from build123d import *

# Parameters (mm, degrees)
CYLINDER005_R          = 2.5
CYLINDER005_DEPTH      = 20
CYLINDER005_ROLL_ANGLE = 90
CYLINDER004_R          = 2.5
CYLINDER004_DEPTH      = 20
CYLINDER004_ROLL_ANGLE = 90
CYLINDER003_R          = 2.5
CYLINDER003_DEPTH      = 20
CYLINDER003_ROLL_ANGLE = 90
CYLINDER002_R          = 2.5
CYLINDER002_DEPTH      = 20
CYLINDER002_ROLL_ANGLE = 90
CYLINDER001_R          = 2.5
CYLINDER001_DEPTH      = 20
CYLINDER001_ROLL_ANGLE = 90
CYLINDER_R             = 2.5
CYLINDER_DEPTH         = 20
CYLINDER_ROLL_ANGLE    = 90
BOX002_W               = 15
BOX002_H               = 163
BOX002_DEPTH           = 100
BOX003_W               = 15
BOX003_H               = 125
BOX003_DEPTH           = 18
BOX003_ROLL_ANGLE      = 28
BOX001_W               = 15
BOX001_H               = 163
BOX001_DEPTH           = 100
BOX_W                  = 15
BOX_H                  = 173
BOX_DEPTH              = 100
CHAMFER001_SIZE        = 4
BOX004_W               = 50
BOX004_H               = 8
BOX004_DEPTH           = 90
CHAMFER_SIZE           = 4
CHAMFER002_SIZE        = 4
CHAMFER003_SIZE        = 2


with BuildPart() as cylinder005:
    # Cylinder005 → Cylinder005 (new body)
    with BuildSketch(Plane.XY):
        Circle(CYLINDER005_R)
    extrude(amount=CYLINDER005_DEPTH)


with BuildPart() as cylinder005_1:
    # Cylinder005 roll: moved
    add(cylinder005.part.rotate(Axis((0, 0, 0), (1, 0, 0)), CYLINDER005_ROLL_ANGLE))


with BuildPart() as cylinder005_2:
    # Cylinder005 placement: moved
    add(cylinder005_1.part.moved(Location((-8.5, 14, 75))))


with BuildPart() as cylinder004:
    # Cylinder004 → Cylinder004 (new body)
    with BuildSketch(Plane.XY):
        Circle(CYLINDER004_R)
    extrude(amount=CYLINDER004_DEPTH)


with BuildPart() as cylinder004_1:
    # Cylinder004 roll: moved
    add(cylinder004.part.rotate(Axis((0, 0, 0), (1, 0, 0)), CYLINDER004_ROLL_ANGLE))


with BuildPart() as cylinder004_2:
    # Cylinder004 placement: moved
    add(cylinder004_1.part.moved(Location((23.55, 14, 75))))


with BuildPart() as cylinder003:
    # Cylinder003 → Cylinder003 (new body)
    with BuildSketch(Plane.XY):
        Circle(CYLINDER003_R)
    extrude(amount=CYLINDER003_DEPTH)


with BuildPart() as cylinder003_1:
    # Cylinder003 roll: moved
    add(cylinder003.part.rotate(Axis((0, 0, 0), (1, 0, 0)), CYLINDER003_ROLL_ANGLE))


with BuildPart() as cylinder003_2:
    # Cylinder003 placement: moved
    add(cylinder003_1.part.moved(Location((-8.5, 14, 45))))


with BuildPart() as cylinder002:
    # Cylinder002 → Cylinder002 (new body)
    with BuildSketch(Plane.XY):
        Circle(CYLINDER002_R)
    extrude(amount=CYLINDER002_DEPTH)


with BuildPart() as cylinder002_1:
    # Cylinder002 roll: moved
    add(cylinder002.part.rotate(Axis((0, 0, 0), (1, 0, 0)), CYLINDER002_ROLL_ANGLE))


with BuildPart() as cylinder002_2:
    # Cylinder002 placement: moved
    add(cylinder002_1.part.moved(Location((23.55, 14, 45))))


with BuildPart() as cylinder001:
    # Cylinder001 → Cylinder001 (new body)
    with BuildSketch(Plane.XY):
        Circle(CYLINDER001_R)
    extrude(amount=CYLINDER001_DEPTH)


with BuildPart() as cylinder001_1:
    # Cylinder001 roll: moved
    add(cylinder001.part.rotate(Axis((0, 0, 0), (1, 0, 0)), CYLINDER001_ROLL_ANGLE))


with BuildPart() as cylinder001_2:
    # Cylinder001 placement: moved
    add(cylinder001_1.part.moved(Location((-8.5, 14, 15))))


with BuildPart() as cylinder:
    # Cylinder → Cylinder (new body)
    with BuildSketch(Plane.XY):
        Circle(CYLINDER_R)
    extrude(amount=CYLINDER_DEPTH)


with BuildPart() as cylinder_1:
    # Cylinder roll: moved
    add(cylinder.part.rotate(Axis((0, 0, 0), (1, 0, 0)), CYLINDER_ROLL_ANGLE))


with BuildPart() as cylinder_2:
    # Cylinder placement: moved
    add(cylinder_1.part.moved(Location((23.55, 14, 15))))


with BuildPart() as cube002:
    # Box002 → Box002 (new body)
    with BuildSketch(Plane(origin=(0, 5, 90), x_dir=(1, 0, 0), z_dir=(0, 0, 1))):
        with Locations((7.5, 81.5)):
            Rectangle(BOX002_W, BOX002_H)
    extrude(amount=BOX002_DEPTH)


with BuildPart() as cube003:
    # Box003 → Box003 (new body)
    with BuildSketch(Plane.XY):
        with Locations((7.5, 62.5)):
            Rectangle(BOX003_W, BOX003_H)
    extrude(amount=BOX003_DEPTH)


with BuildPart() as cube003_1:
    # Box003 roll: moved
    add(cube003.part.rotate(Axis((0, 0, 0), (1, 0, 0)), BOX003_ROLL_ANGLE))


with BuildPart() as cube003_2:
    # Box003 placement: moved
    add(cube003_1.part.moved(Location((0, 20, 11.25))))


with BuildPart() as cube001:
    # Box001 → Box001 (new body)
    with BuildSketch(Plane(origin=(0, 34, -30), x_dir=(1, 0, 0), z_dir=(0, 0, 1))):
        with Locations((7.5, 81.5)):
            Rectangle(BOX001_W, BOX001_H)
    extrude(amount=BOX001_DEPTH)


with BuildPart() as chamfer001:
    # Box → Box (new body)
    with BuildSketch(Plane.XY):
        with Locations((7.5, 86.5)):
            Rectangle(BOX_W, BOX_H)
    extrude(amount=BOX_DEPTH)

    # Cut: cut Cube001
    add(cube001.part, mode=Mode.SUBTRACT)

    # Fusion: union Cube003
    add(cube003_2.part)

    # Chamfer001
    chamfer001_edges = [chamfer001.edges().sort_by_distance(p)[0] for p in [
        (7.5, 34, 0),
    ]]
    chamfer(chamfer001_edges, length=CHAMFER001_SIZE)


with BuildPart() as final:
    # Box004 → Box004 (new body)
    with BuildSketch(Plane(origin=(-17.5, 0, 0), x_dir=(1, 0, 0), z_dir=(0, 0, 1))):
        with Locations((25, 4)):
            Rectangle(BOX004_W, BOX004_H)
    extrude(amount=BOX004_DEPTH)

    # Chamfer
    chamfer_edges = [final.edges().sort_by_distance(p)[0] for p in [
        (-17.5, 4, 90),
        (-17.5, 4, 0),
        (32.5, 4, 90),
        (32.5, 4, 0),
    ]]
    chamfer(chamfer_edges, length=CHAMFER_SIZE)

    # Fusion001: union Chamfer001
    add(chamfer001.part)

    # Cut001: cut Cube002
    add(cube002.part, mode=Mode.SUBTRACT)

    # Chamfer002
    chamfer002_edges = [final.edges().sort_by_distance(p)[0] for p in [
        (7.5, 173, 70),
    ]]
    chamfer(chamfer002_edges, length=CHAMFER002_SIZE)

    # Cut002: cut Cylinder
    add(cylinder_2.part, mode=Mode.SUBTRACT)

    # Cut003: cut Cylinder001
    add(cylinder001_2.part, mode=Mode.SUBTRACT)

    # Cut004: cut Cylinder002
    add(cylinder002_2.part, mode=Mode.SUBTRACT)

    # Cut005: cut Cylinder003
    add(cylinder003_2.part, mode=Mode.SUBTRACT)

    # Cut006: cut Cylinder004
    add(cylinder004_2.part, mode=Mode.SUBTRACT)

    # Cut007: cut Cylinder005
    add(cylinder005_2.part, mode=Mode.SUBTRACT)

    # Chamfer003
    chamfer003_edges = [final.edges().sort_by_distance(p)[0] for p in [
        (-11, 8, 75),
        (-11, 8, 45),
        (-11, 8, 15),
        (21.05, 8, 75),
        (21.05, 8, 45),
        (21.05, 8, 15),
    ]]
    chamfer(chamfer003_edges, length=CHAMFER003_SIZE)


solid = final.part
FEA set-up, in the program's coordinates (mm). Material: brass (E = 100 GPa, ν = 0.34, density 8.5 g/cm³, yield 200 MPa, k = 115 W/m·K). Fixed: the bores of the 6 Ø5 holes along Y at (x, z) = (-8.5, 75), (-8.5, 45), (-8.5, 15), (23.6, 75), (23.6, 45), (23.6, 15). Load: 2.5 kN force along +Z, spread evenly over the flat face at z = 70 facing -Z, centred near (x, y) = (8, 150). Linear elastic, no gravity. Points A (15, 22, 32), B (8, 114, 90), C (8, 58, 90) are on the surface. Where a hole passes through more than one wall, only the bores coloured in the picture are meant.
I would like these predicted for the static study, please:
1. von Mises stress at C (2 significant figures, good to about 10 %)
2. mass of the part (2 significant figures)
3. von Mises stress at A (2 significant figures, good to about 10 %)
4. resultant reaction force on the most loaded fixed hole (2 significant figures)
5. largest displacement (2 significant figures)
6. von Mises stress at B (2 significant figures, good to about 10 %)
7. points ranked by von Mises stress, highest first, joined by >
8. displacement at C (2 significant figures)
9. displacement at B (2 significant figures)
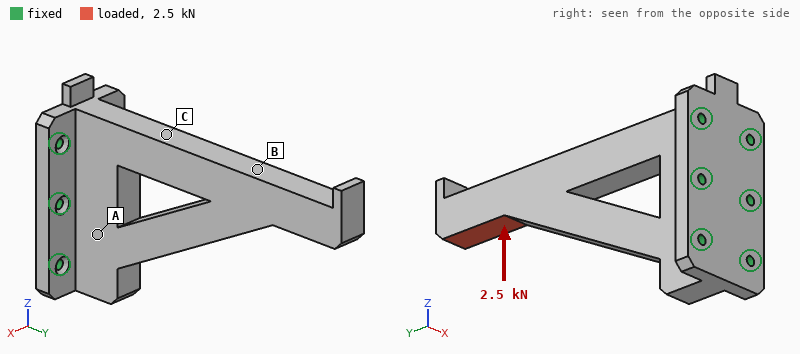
29 MPa
1.2 kg
13 MPa
3.2 kN
0.29 mm
48 MPa
B > C > A
0.044 mm
0.12 mm
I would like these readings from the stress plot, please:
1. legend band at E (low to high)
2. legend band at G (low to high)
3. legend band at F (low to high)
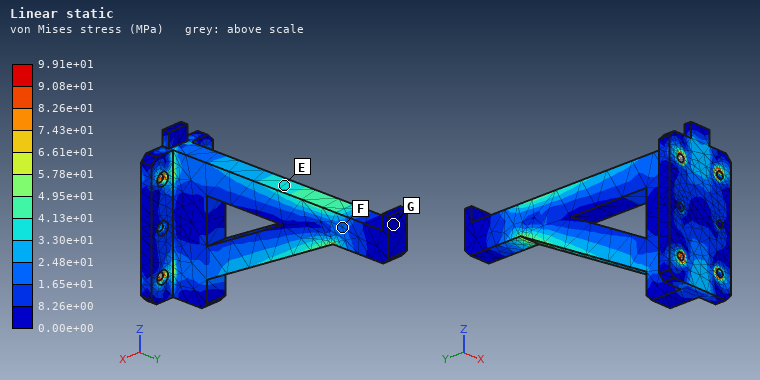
3.30e+01 to 4.13e+01 MPa
0.00e+00 to 8.26e+00 MPa
1.65e+01 to 2.48e+01 MPa
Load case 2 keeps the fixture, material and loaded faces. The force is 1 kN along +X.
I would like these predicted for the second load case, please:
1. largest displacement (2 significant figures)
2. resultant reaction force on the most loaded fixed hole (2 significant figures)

1.1 mm
2.1 kN
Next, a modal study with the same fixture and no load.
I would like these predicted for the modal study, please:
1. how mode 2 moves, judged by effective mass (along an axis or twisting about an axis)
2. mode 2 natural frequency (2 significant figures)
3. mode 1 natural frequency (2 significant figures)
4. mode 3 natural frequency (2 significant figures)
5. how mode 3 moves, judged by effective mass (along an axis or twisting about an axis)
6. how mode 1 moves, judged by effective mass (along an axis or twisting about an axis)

along Z
1300 Hz
390 Hz
1800 Hz
along X
along X
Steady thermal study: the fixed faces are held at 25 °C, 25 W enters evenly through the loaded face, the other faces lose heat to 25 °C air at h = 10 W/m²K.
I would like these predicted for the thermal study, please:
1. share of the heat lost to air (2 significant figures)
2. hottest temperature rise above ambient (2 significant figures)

18 %
60 K
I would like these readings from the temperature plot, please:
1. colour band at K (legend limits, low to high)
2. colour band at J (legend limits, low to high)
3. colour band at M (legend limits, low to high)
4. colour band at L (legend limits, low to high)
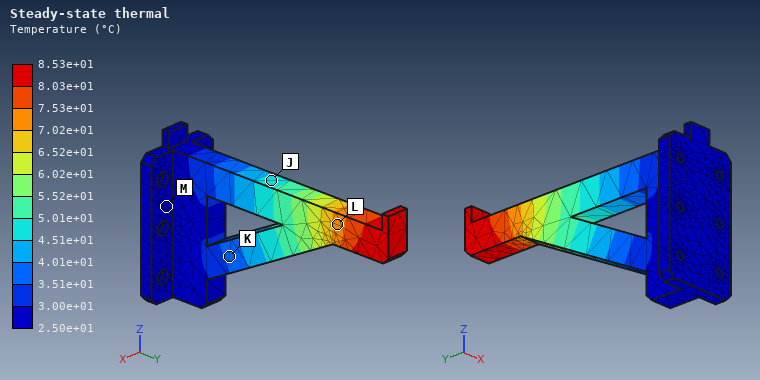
3.51e+01 to 4.01e+01 °C
4.51e+01 to 5.01e+01 °C
2.50e+01 to 3.00e+01 °C
7.02e+01 to 7.53e+01 °C
